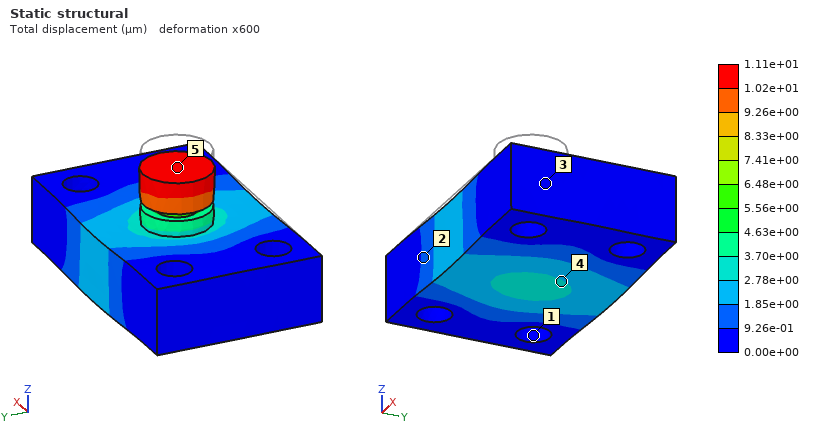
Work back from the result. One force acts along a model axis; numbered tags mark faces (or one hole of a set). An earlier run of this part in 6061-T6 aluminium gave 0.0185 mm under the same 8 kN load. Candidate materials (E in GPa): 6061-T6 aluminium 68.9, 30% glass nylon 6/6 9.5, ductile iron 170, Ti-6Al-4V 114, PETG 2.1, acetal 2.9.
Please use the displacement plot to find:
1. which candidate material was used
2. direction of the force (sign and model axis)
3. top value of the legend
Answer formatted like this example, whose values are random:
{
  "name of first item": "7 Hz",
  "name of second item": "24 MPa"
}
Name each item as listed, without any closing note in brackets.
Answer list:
{
  "which candidate material was used": "Ti-6Al-4V",
  "direction of the force": "-Z",
  "top value of the legend": "1.11e+01 µm"
}
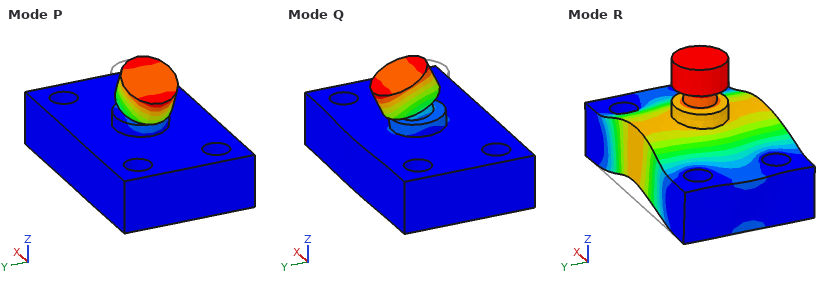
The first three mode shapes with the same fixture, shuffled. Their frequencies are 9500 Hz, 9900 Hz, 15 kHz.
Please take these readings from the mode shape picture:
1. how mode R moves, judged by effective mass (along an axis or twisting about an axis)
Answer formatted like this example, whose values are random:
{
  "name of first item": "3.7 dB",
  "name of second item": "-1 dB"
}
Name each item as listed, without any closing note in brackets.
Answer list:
{
  "how mode R moves, judged by effective mass": "along Z"
}
